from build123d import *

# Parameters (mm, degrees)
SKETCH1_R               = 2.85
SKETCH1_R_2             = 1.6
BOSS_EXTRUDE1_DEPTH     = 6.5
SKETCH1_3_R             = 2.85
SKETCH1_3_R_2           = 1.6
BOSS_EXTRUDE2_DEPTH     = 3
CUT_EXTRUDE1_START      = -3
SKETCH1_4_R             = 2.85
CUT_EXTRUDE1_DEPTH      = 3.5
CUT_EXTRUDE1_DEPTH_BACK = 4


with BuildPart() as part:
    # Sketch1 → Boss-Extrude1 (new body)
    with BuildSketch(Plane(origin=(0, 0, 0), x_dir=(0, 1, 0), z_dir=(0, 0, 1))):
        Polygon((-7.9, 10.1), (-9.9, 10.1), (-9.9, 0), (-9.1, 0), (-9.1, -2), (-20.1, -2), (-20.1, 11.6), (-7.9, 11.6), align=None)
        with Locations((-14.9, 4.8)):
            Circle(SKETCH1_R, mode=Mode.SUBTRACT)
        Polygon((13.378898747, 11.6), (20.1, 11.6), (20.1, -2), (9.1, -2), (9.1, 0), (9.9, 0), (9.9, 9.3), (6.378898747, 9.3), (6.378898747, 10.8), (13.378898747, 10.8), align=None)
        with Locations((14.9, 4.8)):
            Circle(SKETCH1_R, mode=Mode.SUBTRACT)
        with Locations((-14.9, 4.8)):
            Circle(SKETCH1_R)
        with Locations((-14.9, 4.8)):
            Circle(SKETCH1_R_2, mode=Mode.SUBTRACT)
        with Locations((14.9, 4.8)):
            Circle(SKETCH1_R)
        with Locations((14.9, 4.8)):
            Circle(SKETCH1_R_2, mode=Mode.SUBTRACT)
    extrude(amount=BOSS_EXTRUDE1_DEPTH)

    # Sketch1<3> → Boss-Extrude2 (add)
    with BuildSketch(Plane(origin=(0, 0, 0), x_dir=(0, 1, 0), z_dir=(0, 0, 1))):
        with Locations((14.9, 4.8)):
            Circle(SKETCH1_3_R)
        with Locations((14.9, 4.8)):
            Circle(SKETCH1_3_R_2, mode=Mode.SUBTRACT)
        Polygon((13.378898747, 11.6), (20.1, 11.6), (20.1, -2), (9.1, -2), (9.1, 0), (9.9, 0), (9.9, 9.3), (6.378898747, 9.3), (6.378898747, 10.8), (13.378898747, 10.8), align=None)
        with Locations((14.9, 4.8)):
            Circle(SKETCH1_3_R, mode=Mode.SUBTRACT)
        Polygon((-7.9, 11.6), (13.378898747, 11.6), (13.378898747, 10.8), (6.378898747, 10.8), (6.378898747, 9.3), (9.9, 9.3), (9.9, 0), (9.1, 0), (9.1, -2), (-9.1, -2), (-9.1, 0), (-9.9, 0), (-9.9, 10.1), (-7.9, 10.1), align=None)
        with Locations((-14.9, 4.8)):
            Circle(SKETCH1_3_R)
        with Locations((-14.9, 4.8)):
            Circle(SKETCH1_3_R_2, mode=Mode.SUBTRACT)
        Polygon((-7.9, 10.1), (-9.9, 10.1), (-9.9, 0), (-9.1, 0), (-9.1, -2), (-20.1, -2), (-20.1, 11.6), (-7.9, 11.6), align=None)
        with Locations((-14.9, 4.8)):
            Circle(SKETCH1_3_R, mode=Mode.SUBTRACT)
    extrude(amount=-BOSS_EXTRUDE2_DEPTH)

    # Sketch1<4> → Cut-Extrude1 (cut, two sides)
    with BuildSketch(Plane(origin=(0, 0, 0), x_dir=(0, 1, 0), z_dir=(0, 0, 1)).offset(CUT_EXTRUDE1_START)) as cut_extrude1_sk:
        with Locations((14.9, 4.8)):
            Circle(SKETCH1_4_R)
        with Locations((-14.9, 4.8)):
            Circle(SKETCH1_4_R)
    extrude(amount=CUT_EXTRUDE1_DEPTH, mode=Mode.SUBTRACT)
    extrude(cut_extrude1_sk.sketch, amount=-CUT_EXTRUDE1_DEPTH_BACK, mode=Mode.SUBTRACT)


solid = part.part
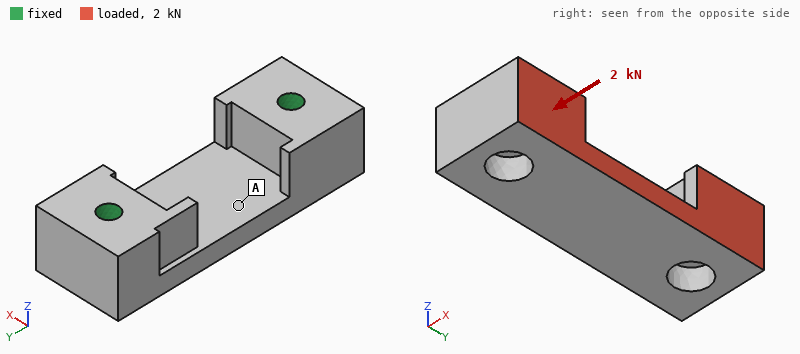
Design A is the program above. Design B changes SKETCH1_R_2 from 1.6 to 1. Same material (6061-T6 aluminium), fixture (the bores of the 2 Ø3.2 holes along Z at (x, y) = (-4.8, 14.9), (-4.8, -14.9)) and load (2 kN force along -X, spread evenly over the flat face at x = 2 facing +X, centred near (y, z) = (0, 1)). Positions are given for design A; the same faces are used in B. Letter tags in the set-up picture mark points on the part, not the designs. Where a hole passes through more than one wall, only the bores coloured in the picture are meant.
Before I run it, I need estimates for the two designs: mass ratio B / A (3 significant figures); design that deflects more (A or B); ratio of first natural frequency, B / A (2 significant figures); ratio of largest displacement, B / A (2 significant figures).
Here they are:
1.02
B
0.86
1.4
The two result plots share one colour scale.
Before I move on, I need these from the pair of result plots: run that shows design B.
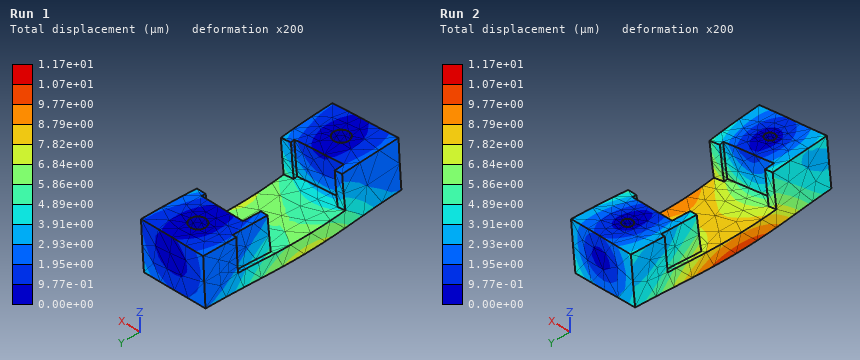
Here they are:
Run 2
